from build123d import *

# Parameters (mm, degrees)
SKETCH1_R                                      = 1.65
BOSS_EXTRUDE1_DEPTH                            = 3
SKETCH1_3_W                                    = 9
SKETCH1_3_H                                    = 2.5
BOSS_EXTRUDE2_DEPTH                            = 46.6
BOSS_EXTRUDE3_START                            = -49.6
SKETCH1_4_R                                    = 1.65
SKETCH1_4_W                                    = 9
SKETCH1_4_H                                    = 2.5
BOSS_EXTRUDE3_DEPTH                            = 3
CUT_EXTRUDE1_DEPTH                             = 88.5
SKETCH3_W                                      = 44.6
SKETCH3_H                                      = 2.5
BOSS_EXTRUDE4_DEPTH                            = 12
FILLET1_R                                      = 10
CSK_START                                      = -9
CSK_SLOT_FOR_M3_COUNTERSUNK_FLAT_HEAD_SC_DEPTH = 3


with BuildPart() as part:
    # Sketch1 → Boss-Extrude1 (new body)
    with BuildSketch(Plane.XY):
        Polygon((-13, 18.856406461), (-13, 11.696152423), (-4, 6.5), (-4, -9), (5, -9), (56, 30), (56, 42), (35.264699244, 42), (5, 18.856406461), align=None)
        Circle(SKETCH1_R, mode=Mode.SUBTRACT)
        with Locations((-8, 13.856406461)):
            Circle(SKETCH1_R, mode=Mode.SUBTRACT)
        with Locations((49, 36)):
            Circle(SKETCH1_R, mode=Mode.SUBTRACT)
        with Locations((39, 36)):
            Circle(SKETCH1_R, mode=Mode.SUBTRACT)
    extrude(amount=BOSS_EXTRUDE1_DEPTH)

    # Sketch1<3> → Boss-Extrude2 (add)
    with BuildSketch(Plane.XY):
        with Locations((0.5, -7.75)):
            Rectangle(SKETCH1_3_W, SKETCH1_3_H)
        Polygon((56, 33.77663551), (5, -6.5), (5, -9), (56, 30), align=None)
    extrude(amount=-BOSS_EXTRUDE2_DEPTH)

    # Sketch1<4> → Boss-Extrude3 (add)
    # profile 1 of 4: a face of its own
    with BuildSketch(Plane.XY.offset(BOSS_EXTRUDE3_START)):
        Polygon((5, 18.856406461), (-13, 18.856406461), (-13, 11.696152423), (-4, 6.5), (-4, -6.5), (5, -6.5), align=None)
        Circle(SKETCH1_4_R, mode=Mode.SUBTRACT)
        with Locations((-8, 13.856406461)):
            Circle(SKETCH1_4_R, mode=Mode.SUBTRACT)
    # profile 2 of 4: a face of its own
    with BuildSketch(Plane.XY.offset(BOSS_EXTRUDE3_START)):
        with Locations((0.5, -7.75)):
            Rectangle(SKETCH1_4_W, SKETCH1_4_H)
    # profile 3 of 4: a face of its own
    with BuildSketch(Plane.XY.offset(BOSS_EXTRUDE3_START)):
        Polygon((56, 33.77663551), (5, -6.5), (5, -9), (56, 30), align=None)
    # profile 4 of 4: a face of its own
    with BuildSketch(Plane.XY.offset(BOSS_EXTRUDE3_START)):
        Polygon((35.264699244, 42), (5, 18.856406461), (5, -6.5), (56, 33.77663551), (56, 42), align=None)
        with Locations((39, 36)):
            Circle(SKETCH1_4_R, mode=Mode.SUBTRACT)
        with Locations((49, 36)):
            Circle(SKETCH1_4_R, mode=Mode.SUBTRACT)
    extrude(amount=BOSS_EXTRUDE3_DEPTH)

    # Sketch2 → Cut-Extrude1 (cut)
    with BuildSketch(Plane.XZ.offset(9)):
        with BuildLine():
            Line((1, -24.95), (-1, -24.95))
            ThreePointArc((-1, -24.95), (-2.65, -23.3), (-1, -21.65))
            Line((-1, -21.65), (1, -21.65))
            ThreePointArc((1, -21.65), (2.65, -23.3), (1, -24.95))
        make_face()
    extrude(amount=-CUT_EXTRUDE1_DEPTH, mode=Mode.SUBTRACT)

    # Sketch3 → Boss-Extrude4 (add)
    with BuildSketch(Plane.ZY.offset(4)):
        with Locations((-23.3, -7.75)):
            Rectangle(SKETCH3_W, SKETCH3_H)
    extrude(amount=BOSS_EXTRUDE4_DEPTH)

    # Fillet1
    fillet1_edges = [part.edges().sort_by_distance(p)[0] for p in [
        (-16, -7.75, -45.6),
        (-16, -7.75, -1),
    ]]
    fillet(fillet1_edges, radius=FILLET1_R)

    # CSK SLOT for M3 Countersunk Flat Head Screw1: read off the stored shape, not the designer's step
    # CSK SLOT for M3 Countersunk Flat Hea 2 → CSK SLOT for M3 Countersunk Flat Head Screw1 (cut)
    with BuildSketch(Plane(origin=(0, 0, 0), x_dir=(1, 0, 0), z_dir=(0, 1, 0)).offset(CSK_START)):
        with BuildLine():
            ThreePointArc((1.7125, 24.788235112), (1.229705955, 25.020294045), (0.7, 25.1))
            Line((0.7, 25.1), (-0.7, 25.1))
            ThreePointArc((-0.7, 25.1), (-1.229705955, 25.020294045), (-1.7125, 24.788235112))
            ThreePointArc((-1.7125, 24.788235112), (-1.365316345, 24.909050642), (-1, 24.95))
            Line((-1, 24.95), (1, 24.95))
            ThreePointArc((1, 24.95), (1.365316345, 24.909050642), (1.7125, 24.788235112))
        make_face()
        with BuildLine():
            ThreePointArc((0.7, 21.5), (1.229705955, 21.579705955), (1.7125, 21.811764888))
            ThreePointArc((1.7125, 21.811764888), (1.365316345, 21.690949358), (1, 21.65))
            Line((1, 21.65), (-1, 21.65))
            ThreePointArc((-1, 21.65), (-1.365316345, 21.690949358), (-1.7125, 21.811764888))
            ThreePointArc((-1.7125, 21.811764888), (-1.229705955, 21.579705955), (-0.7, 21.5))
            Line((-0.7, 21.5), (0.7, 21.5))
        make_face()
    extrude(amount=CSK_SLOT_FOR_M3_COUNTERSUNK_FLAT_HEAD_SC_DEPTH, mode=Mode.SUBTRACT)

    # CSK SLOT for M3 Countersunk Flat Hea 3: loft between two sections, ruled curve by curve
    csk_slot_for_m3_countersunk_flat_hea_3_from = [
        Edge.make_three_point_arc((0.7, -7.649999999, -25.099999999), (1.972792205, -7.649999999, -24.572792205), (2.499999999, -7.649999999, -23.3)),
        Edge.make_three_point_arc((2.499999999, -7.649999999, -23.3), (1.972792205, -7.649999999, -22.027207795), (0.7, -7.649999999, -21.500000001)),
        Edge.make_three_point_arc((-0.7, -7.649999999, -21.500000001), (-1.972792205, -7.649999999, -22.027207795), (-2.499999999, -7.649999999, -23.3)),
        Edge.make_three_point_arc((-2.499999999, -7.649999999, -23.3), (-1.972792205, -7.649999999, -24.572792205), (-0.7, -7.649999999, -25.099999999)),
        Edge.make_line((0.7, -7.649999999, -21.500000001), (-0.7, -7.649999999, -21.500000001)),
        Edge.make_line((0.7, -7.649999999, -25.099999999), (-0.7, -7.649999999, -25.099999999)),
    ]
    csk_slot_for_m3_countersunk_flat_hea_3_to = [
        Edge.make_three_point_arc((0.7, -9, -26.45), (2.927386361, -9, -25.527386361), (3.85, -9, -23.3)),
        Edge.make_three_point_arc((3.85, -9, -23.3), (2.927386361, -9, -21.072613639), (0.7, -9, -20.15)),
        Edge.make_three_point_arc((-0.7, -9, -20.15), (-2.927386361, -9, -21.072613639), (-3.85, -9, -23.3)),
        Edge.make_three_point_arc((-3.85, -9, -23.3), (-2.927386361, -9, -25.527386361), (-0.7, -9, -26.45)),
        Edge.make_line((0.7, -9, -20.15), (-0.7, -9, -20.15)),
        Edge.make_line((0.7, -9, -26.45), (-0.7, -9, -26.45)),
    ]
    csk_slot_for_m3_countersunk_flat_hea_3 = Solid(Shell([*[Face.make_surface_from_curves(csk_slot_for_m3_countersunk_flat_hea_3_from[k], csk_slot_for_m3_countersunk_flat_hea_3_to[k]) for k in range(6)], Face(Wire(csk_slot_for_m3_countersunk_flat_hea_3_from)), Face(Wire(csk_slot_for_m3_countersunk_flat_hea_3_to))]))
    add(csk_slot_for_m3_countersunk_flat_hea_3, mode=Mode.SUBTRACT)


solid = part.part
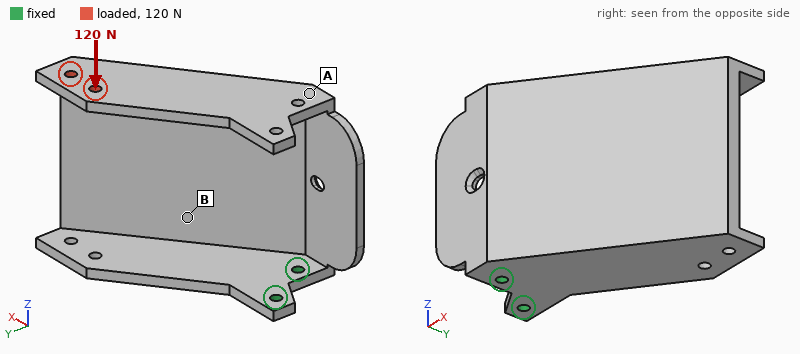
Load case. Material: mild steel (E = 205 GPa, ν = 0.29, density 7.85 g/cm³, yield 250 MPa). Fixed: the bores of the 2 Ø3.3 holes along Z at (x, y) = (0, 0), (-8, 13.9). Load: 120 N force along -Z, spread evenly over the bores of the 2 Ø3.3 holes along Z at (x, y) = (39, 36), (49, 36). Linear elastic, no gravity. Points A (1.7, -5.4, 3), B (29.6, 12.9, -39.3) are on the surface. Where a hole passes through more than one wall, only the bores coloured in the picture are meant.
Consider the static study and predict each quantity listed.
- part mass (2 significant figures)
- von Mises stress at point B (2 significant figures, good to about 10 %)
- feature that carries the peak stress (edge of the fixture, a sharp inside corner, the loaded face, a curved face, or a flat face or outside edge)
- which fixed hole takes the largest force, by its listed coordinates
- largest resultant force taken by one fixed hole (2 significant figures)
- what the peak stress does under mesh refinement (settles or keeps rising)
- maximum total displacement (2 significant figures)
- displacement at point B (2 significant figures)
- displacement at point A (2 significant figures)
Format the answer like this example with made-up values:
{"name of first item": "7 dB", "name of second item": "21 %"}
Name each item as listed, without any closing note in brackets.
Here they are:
{"part mass": "150 g", "von Mises stress at point B": "24 MPa", "feature that carries the peak stress": "edge of the fixture", "which fixed hole takes the largest force, by its listed coordinates": "(0, 0)", "largest resultant force taken by one fixed hole": "100 N", "what the peak stress does under mesh refinement": "keeps rising", "maximum total displacement": "0.29 mm", "displacement at point B": "0.095 mm", "displacement at point A": "0.17 mm"}
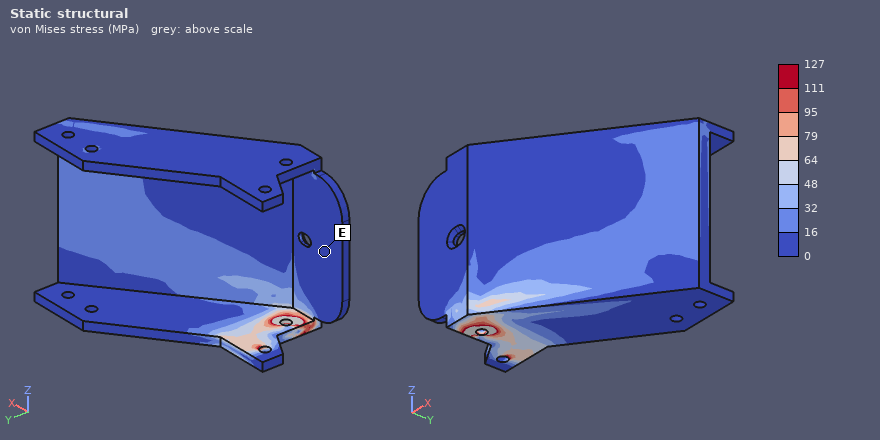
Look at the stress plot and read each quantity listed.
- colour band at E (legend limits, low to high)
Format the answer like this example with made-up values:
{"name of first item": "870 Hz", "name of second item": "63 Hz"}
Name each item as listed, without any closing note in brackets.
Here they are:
{"colour band at E": "0 to 16 MPa"}
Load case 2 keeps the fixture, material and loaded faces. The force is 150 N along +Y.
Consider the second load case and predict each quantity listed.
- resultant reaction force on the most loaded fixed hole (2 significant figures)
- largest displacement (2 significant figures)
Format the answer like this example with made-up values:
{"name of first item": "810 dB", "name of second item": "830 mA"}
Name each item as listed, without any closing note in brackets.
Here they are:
{"resultant reaction force on the most loaded fixed hole": "450 N", "largest displacement": "0.54 mm"}
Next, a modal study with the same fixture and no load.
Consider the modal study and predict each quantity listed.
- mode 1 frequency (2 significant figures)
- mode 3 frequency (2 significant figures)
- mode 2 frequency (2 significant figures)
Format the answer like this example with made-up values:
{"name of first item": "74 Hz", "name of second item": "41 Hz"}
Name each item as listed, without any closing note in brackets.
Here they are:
{"mode 1 frequency": "390 Hz", "mode 3 frequency": "950 Hz", "mode 2 frequency": "410 Hz"}
